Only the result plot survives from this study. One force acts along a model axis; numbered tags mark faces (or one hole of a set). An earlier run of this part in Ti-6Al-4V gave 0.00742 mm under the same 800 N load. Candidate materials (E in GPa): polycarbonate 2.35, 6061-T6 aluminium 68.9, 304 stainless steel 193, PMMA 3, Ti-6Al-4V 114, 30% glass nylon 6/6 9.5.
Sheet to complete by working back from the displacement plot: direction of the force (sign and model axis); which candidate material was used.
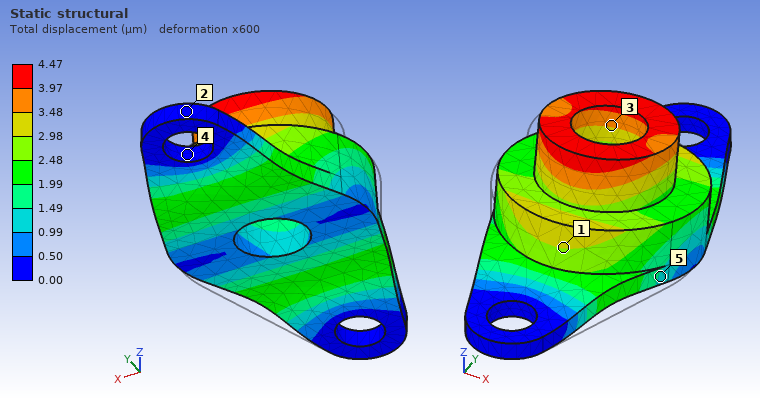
+Y
304 stainless steel
